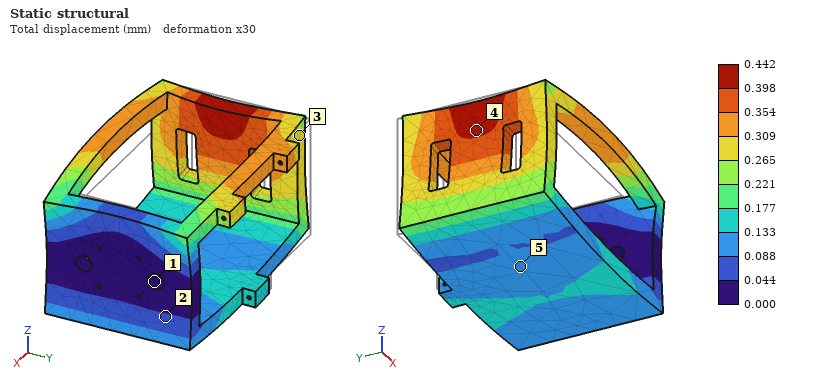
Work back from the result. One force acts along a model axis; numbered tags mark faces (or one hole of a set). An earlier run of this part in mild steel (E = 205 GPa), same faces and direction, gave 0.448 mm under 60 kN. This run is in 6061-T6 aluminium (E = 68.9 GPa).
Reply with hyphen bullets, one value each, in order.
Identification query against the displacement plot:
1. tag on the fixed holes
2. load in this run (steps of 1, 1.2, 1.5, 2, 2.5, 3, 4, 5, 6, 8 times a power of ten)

- 1
- 20 kN
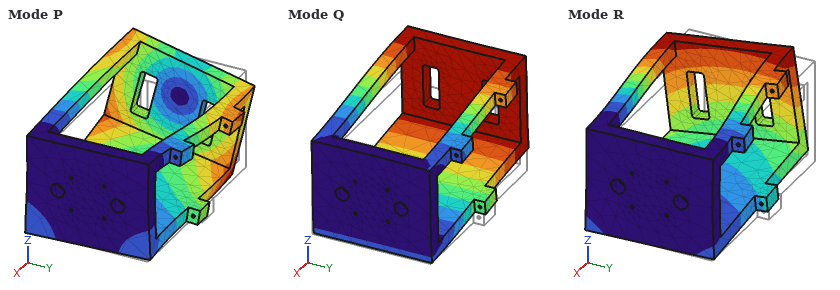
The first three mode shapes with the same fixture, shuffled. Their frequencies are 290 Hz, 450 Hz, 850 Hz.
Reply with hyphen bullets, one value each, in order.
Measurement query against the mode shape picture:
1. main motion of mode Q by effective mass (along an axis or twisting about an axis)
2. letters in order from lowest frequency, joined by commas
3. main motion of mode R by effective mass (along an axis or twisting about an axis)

- along Z
- Q, R, P
- along Y
